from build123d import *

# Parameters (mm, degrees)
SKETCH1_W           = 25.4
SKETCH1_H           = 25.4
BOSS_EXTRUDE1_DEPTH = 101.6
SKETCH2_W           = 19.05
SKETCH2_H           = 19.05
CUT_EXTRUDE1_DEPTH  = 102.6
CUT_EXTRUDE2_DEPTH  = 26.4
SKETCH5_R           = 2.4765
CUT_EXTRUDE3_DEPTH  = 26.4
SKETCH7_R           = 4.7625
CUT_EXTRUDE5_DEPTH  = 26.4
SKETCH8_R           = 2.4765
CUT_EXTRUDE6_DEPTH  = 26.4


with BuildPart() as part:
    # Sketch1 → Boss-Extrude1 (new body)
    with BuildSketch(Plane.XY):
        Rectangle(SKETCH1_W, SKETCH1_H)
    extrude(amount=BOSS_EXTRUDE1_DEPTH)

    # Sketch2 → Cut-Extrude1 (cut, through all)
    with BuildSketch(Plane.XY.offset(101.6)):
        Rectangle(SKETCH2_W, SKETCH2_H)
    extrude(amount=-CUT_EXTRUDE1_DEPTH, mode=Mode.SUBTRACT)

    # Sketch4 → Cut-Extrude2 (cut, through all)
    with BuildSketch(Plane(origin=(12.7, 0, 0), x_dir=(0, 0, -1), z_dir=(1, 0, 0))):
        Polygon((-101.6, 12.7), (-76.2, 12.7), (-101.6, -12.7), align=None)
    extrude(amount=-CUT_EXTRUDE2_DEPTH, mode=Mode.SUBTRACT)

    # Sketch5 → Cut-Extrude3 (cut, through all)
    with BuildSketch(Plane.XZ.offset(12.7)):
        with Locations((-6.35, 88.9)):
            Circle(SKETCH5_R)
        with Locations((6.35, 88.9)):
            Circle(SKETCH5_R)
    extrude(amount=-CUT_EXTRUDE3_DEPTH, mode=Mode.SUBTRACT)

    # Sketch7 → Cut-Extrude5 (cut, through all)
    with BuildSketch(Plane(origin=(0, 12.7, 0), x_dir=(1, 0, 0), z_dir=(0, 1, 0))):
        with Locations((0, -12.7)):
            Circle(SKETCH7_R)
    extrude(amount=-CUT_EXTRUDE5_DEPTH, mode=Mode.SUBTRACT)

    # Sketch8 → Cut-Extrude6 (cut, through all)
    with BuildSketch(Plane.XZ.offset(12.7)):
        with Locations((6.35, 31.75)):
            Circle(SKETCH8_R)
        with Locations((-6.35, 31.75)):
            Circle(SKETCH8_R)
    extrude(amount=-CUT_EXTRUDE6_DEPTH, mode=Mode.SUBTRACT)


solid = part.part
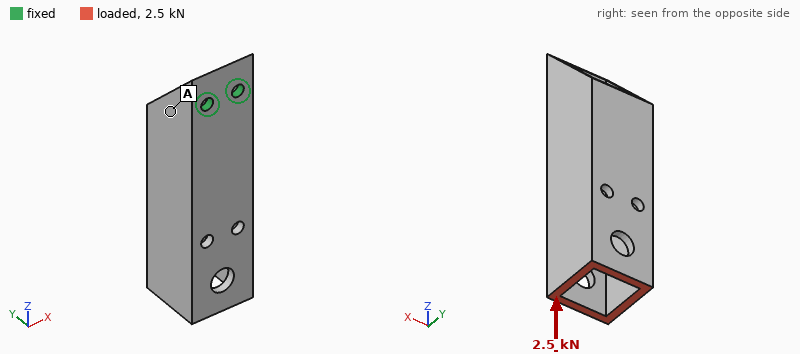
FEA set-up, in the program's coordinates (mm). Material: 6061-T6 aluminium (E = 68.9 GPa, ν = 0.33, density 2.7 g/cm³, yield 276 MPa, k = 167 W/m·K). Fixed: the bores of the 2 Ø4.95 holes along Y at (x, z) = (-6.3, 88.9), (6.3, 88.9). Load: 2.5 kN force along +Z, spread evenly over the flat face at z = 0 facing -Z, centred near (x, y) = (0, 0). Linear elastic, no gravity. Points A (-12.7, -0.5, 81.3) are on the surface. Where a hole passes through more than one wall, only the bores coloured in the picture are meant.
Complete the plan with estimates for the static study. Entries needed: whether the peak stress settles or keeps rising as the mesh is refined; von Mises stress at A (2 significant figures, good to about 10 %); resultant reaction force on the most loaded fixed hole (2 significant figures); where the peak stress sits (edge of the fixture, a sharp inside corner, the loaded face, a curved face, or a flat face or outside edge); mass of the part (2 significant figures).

keeps rising
46 MPa
1.3 kN
edge of the fixture
66 g
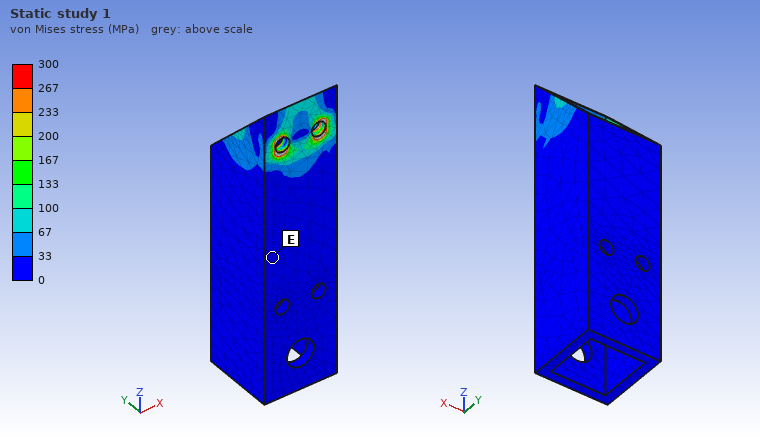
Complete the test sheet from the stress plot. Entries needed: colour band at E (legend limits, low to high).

0 to 33 MPa
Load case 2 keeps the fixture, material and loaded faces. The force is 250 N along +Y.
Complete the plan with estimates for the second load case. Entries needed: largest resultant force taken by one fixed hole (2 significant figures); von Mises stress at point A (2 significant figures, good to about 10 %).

130 N
34 MPa
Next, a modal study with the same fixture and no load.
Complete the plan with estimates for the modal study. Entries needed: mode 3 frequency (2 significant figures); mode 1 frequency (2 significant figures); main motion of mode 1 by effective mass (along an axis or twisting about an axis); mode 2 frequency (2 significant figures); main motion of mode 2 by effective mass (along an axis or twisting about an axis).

2700 Hz
690 Hz
along Y
1700 Hz
along X
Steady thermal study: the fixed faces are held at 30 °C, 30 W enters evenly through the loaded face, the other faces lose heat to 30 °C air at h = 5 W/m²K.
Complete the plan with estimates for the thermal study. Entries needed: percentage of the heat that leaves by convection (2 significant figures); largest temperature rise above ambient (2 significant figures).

9.9 %
69 K
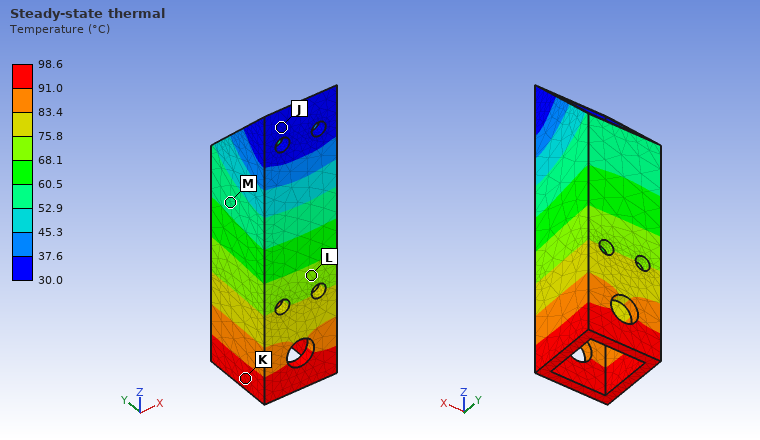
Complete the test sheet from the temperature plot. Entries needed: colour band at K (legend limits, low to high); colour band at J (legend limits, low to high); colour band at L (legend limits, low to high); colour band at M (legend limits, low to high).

91.0 to 98.6 °C
30.0 to 37.6 °C
68.1 to 75.8 °C
52.9 to 60.5 °C
